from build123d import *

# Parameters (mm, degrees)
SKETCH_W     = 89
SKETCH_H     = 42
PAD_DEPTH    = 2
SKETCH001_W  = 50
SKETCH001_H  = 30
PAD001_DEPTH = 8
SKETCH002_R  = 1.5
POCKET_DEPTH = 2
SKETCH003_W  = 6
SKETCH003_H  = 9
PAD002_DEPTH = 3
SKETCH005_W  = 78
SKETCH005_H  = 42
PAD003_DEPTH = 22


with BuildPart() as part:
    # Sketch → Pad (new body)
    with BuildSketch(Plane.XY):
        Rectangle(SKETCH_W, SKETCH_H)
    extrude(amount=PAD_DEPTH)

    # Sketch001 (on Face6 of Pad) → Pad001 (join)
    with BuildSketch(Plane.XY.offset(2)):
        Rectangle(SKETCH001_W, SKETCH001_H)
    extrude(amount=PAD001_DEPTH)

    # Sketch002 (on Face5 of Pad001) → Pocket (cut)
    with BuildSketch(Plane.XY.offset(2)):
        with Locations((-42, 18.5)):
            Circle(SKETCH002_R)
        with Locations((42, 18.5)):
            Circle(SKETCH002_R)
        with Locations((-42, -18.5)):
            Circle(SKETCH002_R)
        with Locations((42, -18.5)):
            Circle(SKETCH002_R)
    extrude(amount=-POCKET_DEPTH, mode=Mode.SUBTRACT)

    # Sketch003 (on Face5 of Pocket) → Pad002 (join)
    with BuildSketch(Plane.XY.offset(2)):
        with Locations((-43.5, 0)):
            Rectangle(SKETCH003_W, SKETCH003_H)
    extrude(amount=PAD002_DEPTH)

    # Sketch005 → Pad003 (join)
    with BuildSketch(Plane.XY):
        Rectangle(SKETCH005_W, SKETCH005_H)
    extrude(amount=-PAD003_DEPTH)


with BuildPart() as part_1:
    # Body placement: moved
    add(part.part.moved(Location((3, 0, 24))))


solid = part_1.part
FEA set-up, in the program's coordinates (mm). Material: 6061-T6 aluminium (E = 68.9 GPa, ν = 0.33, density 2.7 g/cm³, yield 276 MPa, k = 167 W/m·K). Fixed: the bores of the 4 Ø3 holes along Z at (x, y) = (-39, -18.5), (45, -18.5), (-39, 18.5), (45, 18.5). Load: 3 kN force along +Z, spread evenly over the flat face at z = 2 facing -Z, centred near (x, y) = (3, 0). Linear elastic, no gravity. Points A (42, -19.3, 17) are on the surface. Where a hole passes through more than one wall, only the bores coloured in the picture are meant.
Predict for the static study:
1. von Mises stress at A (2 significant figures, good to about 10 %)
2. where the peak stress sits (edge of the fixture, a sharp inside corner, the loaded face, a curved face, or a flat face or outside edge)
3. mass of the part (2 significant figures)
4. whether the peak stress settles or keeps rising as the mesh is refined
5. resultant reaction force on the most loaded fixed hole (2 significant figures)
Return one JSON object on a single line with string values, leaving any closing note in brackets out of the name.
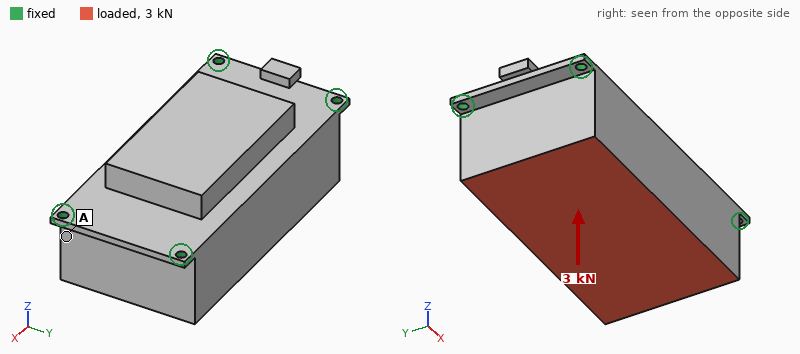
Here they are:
{"von Mises stress at A": "13 MPa", "where the peak stress sits": "edge of the fixture", "mass of the part": "250 g", "whether the peak stress settles or keeps rising as the mesh is refined": "keeps rising", "resultant reaction force on the most loaded fixed hole": "870 N"}
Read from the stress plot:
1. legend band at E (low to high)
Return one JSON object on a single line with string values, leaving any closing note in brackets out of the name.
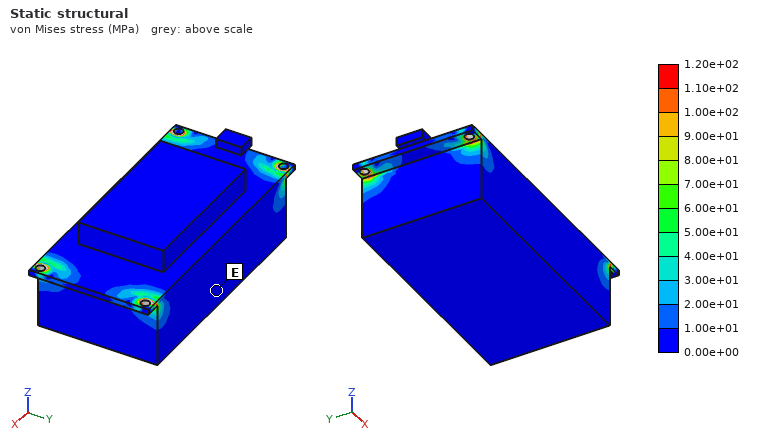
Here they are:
{"legend band at E": "0.00e+00 to 1.00e+01 MPa"}
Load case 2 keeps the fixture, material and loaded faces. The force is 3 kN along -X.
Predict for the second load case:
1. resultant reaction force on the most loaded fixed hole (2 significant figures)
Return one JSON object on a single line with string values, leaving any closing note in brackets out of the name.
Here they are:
{"resultant reaction force on the most loaded fixed hole": "890 N"}
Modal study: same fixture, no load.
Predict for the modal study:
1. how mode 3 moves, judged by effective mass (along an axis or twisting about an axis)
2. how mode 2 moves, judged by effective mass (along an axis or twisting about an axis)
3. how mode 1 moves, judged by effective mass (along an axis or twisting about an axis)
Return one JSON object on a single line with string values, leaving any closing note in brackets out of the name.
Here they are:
{"how mode 3 moves, judged by effective mass": "along X", "how mode 2 moves, judged by effective mass": "along Y", "how mode 1 moves, judged by effective mass": "along Z"}
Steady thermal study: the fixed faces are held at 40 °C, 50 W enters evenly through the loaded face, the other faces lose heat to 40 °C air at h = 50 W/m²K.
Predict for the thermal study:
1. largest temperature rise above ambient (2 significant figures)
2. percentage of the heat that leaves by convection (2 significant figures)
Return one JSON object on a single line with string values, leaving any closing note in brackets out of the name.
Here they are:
{"largest temperature rise above ambient": "20 K", "percentage of the heat that leaves by convection": "20 %"}
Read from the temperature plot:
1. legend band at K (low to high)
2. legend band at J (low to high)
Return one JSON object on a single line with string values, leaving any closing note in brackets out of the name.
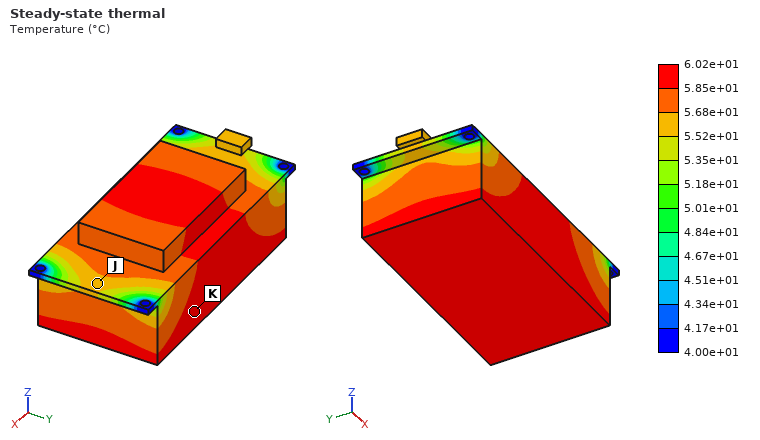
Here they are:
{"legend band at K": "5.85e+01 to 6.02e+01 °C", "legend band at J": "5.52e+01 to 5.68e+01 °C"}
